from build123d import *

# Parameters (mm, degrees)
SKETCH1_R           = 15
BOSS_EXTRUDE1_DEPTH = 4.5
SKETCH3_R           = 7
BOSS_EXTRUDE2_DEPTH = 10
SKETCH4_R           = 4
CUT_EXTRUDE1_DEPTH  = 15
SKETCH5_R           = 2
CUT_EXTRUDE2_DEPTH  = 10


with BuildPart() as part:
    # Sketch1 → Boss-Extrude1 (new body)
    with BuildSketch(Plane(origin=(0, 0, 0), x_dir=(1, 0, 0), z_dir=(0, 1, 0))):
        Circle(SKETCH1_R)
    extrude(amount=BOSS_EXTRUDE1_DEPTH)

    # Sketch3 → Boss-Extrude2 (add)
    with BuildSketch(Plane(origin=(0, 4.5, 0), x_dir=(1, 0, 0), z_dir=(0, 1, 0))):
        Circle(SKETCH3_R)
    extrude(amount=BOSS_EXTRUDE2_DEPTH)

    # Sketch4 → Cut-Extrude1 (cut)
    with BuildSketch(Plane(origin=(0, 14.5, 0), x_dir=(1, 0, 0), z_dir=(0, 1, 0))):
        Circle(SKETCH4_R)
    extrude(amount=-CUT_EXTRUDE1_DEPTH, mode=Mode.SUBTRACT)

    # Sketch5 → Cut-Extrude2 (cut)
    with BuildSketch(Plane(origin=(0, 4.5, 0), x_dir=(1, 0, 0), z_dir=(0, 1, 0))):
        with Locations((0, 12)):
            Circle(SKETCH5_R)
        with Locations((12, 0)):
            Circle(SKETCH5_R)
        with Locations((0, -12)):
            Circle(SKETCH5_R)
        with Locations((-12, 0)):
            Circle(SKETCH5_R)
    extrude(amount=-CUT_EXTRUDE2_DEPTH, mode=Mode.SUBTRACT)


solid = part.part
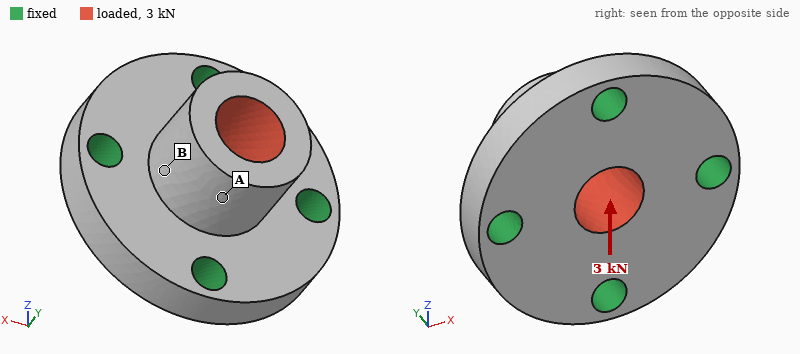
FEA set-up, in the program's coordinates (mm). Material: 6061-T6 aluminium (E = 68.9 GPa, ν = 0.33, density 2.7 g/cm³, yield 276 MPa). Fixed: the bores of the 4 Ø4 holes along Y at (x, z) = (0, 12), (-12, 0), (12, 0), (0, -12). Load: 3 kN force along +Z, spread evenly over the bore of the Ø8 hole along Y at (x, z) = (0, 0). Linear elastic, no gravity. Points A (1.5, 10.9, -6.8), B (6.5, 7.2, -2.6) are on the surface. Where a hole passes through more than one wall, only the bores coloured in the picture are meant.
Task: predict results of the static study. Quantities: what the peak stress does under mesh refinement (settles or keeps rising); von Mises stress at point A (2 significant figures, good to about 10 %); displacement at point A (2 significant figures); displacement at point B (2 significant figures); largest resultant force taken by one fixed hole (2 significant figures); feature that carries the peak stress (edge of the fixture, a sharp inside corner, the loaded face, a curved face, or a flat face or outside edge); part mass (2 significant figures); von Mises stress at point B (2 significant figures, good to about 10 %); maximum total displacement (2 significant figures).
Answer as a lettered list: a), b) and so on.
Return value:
a) keeps rising
b) 11 MPa
c) 15 µm
d) 7.9 µm
e) 1.2 kN
f) edge of the fixture
g) 10 g
h) 29 MPa
i) 20 µm
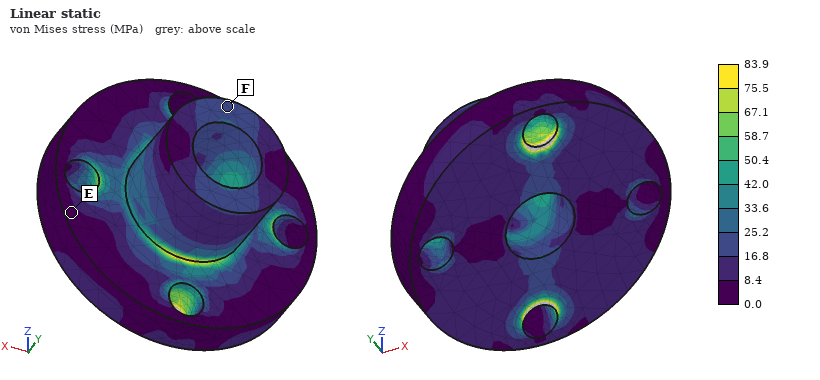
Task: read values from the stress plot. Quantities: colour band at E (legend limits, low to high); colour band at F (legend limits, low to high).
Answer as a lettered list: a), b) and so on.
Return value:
a) 0.0 to 8.4 MPa
b) 16.8 to 25.2 MPa
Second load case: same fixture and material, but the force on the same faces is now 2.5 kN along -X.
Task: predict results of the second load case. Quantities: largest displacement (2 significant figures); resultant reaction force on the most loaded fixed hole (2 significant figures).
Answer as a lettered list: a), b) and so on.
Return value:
a) 17 µm
b) 1.0 kN
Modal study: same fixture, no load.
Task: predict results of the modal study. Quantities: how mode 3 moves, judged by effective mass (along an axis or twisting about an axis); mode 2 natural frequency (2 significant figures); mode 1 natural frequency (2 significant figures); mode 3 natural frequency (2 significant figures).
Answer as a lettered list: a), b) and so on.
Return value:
a) along Y
b) 35 kHz
c) 35 kHz
d) 46 kHz
